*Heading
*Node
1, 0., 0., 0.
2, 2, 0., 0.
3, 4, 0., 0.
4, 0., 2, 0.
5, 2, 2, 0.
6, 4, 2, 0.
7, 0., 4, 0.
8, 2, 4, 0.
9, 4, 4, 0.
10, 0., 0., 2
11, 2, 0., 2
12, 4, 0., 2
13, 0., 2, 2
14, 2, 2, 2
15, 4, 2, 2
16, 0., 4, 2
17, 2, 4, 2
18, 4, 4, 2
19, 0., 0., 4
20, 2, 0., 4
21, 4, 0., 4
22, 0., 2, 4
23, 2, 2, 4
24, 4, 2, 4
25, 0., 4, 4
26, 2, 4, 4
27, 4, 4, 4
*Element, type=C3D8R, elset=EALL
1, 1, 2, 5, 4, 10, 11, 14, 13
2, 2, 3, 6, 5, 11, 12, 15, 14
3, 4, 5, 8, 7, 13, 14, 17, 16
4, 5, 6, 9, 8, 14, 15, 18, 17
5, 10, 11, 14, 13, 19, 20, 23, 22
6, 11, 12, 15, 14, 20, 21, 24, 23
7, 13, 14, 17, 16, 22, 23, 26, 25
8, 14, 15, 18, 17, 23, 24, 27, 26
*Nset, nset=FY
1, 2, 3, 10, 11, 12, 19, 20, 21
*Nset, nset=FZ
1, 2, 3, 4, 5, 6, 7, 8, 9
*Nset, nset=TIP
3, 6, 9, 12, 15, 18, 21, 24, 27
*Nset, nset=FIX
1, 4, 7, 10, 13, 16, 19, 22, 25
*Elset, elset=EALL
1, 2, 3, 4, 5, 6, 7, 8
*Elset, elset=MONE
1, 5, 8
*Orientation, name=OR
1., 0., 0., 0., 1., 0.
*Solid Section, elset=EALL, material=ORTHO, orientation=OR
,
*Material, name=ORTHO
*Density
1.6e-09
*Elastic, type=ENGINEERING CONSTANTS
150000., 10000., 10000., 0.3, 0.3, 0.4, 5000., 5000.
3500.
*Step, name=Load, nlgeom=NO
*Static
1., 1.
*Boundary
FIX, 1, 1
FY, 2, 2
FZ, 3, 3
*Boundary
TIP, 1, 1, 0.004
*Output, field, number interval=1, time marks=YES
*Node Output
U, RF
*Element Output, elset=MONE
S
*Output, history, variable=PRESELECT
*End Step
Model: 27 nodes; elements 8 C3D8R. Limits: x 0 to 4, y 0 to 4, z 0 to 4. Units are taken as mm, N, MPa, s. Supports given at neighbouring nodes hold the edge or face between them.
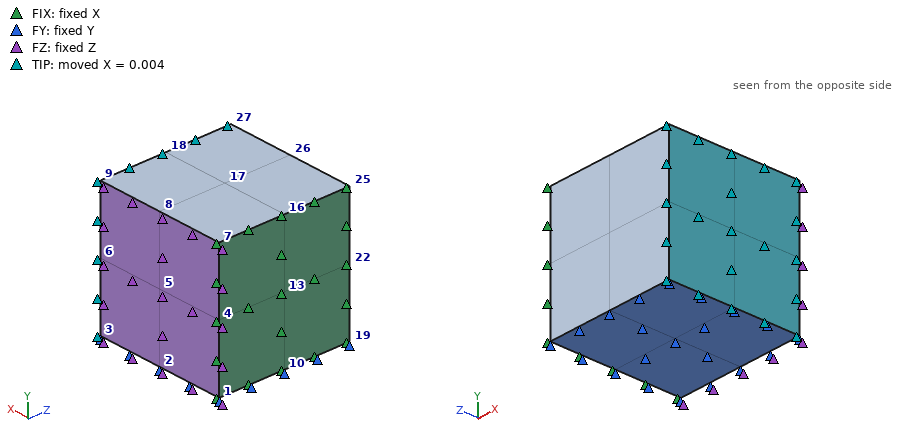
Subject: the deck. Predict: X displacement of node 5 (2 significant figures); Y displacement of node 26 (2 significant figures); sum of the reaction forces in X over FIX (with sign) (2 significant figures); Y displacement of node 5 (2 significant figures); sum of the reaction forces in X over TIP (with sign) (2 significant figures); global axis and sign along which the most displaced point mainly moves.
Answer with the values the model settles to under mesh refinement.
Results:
0.0020 mm
-0.0012 mm
-2400 N
-6.0e-04 mm
2400 N
+X
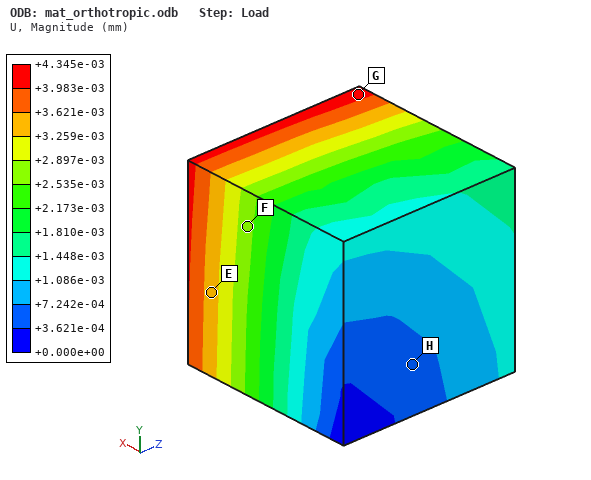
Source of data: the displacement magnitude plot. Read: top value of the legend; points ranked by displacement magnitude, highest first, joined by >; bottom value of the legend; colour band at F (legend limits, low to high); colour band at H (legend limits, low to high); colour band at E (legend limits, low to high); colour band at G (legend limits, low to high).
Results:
+4.345e-03 mm
G > E > F > H
+0.000e+00 mm
+2.535e-03 to +2.897e-03 mm
+3.621e-04 to +7.242e-04 mm
+3.259e-03 to +3.621e-03 mm
+3.983e-03 to +4.345e-03 mm
